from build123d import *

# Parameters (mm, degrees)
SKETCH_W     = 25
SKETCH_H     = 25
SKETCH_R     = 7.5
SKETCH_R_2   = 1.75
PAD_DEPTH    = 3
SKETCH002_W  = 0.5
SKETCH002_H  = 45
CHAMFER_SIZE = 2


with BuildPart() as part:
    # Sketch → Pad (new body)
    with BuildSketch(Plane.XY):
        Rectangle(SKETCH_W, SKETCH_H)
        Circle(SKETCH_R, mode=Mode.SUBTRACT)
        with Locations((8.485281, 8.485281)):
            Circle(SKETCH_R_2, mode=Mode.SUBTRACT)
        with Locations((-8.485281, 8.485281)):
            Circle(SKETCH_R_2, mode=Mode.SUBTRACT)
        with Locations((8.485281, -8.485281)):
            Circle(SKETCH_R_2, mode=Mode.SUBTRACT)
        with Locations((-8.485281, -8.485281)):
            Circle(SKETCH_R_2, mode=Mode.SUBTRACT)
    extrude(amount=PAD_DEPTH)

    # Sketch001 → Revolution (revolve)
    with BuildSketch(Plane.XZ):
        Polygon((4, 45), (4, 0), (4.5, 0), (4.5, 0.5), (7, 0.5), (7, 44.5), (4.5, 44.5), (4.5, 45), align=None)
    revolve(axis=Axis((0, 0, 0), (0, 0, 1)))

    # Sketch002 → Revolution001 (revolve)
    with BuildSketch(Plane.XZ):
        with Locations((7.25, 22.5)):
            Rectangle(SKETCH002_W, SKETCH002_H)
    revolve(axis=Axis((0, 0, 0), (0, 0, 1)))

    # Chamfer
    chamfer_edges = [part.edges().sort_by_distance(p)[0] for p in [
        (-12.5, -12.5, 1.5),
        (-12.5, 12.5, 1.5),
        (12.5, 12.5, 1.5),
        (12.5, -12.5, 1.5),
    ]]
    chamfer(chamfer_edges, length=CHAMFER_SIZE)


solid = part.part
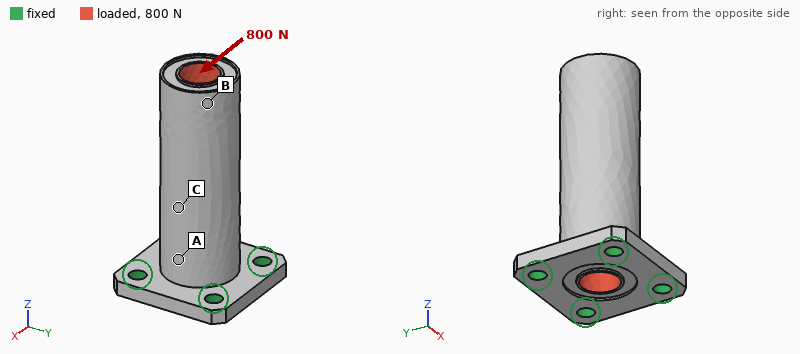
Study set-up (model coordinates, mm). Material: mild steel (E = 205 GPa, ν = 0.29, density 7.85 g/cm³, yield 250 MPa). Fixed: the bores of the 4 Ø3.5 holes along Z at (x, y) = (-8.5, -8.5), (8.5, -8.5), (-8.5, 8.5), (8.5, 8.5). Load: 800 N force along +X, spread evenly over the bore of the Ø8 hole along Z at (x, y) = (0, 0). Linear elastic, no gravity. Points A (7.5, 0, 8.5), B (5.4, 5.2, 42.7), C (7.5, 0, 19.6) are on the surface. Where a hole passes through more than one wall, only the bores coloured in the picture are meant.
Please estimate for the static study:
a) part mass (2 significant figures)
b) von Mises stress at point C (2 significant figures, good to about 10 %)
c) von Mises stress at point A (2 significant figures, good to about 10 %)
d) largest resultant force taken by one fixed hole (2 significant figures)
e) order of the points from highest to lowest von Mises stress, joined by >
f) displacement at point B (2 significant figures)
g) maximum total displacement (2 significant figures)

53 g
19 MPa
36 MPa
640 N
A > C > B
37 µm
40 µm
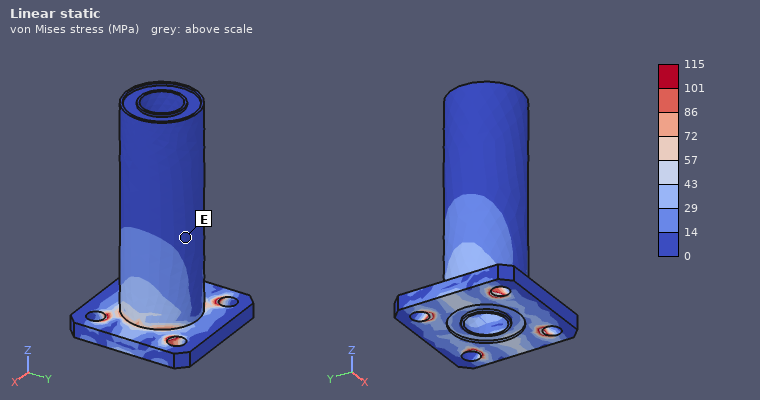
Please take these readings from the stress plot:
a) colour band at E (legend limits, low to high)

0 to 14 MPa
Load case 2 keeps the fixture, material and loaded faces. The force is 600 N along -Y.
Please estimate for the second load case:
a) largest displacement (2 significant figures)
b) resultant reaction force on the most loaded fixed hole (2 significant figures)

30 µm
480 N
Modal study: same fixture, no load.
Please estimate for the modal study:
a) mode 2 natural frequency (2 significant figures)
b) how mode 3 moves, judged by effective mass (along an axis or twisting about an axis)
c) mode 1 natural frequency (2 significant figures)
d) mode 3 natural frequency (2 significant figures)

4200 Hz
along Z
4200 Hz
18 kHz
